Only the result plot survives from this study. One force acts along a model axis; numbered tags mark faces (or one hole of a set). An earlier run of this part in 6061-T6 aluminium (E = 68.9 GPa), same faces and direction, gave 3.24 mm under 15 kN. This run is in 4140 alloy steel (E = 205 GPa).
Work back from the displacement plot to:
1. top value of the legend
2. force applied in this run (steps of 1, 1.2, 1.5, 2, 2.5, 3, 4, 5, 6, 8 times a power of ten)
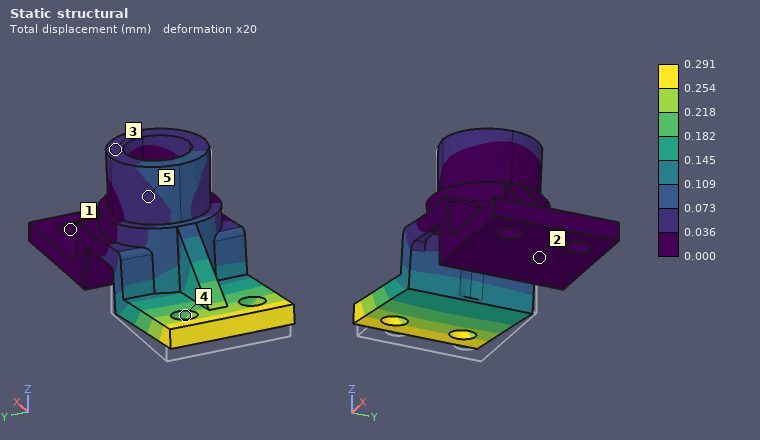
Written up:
0.291 mm
4 kN
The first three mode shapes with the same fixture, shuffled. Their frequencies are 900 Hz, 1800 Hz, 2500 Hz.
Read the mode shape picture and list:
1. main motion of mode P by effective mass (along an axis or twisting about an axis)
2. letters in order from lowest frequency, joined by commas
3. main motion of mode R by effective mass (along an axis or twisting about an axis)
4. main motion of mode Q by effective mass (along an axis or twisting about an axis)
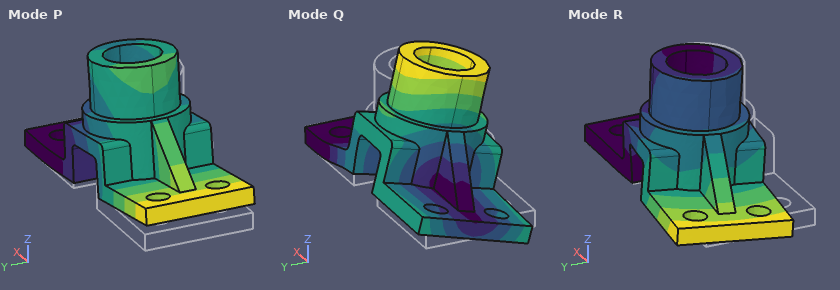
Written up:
along Z
P, R, Q
along Y
along Y
